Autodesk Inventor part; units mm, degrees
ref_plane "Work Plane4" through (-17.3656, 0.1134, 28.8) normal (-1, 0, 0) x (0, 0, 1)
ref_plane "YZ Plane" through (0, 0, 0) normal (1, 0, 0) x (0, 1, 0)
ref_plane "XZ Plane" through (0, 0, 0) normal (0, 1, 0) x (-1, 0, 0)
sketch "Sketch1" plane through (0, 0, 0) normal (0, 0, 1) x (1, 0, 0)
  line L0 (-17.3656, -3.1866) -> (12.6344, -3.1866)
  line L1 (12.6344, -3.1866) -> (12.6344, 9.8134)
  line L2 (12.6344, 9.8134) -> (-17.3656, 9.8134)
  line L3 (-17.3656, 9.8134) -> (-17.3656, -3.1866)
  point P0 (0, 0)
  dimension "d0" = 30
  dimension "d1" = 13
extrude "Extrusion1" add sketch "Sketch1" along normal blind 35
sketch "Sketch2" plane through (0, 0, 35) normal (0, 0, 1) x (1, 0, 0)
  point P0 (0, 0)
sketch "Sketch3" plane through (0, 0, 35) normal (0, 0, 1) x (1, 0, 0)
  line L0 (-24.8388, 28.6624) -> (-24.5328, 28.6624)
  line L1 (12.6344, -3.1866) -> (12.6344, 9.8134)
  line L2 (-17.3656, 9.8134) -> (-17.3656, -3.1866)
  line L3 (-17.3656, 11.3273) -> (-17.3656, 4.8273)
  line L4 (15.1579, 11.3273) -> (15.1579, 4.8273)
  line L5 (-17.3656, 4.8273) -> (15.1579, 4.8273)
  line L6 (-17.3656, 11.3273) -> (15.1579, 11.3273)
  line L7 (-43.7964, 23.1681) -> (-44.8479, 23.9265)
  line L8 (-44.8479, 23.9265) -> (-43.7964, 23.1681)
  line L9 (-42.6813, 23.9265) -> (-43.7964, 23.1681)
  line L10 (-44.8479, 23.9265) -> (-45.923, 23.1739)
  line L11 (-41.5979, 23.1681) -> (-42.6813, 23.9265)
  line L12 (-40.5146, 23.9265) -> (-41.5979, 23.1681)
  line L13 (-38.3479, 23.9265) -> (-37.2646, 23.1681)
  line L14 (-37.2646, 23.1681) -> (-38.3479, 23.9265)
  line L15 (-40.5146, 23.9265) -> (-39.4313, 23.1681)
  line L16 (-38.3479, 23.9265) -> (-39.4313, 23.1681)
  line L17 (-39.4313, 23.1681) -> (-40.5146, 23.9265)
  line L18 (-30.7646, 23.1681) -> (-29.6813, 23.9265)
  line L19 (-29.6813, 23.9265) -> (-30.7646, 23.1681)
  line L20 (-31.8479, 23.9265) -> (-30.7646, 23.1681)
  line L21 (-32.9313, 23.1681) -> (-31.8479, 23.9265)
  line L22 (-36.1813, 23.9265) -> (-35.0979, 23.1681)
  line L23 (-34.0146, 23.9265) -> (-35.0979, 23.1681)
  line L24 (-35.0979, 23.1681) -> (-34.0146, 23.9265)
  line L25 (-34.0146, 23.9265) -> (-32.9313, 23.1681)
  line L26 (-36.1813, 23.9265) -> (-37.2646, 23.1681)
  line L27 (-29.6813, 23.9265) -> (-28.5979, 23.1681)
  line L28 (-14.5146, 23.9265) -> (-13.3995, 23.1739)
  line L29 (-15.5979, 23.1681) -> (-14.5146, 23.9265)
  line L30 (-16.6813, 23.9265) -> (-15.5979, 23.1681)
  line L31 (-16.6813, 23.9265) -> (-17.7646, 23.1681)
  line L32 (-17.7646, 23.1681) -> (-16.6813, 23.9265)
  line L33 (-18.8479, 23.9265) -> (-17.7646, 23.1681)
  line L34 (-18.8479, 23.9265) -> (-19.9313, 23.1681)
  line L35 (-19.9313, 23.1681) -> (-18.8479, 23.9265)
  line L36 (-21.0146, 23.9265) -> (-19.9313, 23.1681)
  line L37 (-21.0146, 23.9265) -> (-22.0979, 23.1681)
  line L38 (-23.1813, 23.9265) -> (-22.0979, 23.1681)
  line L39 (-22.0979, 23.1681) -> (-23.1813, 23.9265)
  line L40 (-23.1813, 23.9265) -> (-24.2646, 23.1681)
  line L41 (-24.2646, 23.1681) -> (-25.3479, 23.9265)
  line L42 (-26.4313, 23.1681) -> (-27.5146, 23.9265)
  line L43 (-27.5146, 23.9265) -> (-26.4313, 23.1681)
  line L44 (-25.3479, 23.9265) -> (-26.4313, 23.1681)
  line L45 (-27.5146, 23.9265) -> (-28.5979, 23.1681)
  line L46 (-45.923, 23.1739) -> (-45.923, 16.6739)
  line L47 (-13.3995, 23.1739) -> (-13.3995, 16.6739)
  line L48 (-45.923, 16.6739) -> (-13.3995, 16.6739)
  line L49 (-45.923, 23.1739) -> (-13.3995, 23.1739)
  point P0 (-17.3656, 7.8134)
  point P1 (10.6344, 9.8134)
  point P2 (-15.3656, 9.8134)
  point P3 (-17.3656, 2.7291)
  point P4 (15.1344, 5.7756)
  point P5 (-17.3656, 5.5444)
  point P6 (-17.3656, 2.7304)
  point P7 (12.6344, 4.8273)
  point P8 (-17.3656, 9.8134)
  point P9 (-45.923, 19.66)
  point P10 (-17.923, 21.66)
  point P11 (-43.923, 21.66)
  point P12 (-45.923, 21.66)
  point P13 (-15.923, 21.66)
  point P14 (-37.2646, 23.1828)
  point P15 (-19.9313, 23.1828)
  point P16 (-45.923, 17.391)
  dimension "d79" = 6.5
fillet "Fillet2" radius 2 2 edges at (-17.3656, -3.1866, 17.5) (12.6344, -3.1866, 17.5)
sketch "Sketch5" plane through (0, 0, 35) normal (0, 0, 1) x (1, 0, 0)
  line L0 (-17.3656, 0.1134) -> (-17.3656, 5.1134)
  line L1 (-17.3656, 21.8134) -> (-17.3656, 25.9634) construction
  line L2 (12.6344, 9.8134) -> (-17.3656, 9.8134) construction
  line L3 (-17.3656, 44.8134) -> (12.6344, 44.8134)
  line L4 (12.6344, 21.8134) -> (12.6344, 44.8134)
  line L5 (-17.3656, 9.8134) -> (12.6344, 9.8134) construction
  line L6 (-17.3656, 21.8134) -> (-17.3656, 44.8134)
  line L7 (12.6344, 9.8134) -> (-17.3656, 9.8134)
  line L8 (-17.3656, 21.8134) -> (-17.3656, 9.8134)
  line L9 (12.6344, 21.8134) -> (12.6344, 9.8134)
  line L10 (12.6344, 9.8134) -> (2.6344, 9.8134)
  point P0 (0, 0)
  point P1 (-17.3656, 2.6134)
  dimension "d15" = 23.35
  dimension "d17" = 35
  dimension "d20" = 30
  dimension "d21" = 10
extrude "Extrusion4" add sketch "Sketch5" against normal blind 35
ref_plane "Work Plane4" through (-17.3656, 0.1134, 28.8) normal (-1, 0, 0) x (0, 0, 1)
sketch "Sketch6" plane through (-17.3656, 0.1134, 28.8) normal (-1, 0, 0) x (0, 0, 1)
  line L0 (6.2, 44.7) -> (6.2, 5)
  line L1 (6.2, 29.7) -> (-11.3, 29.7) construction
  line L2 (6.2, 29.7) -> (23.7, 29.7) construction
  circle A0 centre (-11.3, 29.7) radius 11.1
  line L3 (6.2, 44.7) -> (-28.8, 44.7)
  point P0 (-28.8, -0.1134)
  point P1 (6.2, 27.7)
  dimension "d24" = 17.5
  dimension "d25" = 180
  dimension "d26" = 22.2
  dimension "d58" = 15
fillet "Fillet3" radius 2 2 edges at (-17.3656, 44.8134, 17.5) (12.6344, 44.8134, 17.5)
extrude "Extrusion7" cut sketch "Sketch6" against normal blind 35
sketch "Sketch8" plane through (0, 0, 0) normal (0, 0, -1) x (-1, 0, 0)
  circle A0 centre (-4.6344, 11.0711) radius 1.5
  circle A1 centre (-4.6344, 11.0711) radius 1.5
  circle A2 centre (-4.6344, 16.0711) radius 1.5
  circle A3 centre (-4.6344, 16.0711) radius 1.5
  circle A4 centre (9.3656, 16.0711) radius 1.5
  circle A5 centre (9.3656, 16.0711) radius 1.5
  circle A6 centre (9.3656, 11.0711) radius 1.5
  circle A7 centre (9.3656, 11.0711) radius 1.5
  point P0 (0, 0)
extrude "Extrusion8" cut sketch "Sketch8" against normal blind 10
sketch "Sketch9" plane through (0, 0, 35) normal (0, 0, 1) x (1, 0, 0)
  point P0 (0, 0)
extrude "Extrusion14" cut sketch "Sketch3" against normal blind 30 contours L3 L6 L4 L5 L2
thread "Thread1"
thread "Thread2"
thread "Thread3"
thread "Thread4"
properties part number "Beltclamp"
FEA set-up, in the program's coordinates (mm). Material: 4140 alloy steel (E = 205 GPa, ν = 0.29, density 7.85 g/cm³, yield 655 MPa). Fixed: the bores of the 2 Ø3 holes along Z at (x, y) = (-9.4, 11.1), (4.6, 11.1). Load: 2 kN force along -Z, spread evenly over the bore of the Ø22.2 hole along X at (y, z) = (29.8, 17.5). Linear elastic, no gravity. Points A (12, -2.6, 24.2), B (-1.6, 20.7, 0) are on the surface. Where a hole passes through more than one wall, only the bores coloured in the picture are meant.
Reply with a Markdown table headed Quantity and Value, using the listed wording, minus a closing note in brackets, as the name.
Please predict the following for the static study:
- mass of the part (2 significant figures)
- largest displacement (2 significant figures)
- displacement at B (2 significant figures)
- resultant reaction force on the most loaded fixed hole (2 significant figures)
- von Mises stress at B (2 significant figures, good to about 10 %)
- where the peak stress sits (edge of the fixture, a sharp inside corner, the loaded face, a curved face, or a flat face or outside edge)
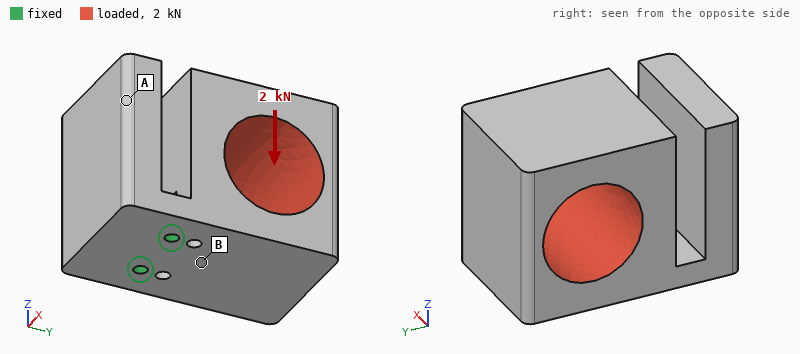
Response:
| Quantity | Value |
|---|---|
| mass of the part | 260 g |
| largest displacement | 39 µm |
| displacement at B | 6.6 µm |
| resultant reaction force on the most loaded fixed hole | 1.0 kN |
| von Mises stress at B | 30 MPa |
| where the peak stress sits | a flat face or outside edge |
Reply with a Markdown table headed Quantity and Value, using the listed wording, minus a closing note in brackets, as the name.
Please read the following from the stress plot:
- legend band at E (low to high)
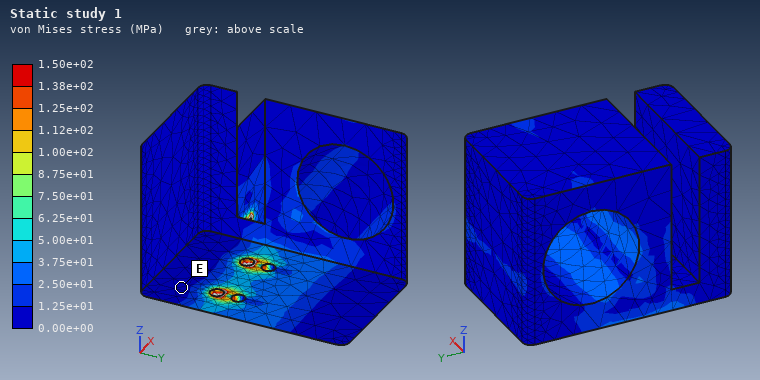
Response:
| Quantity | Value |
|---|---|
| legend band at E | 0.00e+00 to 1.25e+01 MPa |
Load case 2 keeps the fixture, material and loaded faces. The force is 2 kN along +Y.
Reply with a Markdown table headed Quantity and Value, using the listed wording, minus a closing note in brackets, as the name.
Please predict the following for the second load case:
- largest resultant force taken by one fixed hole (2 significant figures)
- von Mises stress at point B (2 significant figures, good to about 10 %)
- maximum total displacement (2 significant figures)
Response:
| Quantity | Value |
|---|---|
| largest resultant force taken by one fixed hole | 1.0 kN |
| von Mises stress at point B | 11 MPa |
| maximum total displacement | 29 µm |
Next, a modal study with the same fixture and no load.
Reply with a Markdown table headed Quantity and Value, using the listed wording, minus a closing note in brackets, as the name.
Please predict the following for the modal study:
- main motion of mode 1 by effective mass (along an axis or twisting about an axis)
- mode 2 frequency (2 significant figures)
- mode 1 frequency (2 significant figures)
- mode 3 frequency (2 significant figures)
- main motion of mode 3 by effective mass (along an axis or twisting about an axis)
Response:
| Quantity | Value |
|---|---|
| main motion of mode 1 by effective mass | along Y |
| mode 2 frequency | 2900 Hz |
| mode 1 frequency | 2600 Hz |
| mode 3 frequency | 5500 Hz |
| main motion of mode 3 by effective mass | along X |
